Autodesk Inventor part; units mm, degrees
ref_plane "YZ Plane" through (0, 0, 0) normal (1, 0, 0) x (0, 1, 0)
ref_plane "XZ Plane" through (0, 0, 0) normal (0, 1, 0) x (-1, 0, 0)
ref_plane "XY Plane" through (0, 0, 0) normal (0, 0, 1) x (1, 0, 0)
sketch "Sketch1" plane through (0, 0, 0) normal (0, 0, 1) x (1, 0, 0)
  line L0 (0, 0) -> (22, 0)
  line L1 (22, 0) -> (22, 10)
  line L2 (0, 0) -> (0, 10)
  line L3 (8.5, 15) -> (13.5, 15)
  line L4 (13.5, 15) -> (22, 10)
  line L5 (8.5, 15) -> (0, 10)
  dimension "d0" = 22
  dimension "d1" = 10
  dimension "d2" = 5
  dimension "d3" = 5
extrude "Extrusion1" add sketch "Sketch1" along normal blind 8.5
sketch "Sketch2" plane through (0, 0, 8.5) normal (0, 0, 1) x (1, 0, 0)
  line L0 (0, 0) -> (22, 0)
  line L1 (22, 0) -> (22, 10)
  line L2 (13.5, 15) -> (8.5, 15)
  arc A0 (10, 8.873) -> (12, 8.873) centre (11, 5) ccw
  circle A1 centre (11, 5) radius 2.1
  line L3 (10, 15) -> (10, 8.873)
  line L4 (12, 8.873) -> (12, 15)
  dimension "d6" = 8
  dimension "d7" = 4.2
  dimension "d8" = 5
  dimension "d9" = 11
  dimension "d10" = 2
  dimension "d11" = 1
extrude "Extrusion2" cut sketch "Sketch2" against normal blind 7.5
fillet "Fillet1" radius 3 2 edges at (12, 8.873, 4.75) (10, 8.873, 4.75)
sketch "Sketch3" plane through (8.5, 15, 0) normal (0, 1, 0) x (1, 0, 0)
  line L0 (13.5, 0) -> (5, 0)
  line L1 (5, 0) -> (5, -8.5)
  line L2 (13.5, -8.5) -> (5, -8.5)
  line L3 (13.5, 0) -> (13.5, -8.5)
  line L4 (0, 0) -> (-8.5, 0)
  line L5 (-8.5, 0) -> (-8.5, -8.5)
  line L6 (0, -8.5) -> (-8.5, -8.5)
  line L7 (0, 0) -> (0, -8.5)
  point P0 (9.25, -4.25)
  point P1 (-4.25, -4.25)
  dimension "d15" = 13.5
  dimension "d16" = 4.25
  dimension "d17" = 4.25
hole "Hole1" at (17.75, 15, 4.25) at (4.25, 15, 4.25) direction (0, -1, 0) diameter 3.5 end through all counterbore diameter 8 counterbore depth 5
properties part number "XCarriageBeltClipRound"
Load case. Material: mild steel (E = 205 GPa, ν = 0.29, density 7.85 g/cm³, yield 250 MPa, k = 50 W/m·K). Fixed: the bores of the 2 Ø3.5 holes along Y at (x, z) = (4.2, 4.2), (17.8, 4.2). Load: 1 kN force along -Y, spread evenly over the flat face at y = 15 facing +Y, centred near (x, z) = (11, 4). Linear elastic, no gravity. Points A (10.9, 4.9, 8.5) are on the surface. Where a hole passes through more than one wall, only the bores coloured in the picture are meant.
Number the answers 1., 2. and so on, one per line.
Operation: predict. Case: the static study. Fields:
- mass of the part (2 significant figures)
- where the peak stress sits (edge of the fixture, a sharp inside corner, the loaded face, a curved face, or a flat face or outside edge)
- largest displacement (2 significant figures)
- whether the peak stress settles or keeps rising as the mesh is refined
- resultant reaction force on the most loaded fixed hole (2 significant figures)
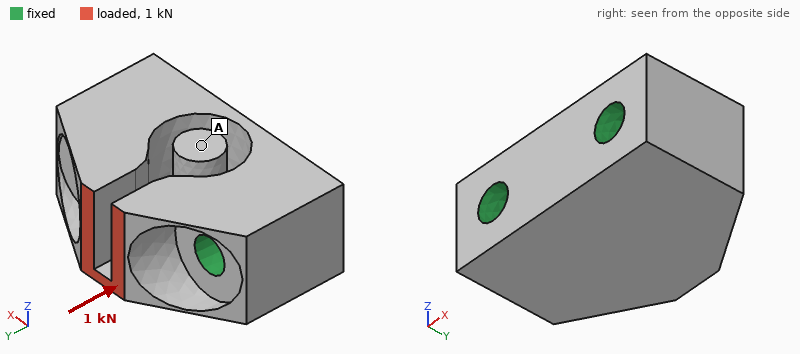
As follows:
1. 13 g
2. a sharp inside corner
3. 4.8 µm
4. keeps rising
5. 510 N
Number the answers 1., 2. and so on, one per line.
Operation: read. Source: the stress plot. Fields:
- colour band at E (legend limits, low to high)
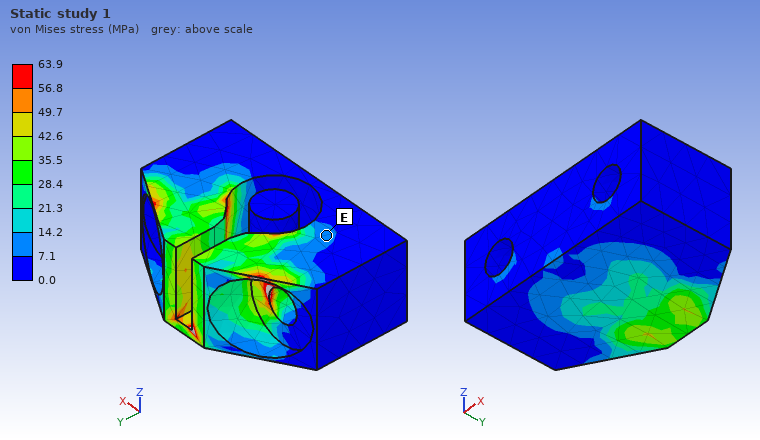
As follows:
1. 7.1 to 14.2 MPa
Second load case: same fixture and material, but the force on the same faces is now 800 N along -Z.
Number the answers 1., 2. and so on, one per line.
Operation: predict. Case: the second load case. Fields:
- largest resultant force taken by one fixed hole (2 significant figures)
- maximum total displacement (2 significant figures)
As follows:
1. 400 N
2. 8.4 µm
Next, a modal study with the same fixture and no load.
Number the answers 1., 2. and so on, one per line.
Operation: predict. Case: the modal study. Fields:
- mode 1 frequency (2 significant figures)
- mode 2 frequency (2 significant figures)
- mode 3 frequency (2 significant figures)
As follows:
1. 25 kHz
2. 26 kHz
3. 51 kHz
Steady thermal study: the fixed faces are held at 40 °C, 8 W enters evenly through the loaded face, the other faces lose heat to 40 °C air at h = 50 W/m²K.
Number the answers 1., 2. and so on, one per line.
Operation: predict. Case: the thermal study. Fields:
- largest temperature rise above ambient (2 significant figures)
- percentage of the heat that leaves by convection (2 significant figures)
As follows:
1. 30 K
2. 4.5 %
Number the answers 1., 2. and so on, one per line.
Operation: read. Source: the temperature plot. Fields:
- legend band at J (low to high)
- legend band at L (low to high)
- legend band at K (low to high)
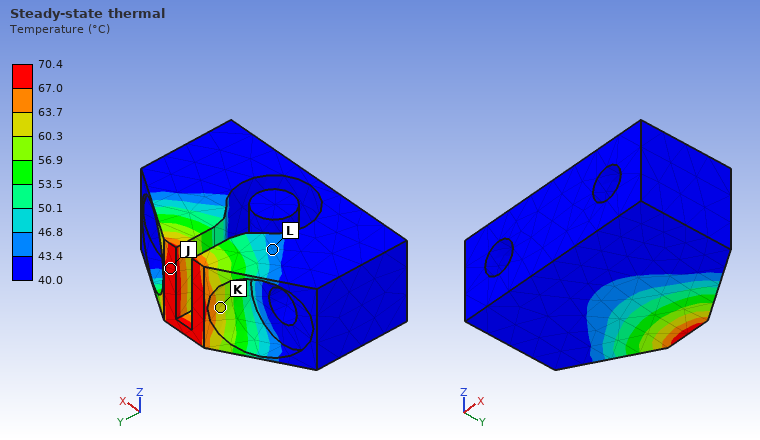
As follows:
1. 67.0 to 70.4 °C
2. 43.4 to 46.8 °C
3. 60.3 to 63.7 °C
